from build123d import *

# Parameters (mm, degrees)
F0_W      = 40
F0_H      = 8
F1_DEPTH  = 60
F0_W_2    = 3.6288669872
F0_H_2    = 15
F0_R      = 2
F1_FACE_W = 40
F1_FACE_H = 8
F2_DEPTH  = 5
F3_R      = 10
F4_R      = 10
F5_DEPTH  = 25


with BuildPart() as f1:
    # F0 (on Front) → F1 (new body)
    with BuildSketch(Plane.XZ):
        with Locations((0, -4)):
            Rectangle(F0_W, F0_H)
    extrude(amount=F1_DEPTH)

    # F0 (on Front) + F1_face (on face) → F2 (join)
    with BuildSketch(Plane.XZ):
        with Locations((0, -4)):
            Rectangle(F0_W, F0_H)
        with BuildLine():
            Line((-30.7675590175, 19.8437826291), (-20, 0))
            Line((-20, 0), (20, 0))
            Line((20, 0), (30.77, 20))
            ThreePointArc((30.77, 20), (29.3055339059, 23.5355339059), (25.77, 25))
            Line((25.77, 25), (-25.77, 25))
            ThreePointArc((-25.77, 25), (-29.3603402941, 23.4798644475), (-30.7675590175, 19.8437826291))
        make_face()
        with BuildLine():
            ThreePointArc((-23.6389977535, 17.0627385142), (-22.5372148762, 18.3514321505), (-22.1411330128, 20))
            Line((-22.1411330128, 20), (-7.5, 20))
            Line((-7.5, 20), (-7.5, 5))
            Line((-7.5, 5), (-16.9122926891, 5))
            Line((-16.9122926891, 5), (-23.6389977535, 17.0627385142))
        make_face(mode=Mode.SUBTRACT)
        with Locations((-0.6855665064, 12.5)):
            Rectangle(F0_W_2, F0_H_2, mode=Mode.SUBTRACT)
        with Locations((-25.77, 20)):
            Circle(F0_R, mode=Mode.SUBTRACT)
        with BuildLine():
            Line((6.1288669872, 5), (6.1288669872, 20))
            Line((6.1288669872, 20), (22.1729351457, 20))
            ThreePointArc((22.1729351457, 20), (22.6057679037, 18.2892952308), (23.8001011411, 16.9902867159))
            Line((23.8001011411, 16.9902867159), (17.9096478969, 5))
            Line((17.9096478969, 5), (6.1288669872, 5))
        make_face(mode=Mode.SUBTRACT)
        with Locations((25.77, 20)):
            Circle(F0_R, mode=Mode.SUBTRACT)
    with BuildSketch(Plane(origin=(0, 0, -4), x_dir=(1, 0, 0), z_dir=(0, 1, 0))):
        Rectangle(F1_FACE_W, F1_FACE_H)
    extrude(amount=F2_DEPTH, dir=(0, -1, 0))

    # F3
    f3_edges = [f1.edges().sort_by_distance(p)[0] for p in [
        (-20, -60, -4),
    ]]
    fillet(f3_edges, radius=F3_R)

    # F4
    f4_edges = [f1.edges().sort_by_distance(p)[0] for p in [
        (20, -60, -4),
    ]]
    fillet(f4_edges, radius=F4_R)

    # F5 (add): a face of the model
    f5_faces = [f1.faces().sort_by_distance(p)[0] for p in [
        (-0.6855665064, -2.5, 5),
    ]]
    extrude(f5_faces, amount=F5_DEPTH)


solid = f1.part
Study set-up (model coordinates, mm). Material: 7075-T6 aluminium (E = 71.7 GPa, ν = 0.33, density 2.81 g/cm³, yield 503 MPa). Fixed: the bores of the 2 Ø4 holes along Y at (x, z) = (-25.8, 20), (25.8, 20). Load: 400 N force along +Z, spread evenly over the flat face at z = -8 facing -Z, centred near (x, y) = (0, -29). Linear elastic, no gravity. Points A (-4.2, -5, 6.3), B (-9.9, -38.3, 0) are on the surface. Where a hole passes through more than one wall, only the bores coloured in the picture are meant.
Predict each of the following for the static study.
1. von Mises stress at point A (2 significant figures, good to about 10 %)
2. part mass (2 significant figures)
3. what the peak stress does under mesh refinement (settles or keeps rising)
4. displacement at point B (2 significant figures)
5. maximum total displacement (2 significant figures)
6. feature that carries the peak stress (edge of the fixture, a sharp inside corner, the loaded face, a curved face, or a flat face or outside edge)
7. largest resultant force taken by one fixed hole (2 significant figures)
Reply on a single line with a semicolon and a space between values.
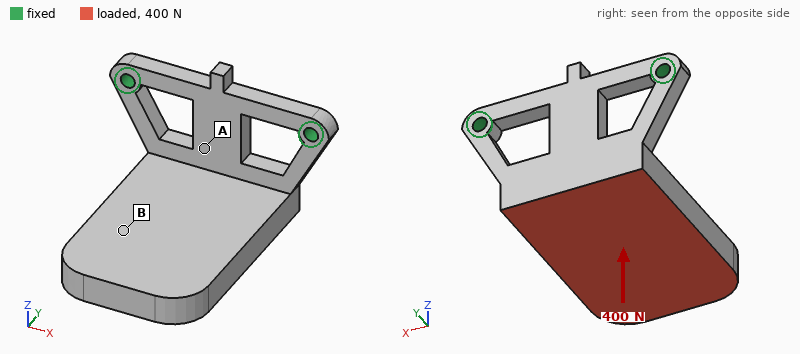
99 MPa; 65 g; keeps rising; 0.65 mm; 1.1 mm; edge of the fixture; 220 N
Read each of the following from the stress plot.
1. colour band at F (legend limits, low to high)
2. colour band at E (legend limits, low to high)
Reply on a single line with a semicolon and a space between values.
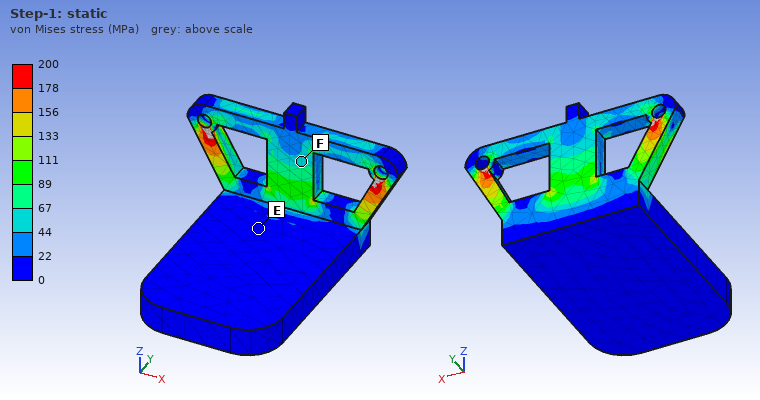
44 to 67 MPa; 0 to 22 MPa
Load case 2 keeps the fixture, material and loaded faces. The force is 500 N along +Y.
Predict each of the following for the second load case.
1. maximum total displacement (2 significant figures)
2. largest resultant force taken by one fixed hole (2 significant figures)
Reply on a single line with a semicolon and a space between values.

0.91 mm; 250 N
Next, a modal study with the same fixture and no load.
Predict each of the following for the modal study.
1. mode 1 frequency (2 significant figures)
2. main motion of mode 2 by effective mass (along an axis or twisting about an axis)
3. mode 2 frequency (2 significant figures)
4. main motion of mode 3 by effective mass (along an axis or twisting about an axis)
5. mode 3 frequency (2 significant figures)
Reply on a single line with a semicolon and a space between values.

490 Hz; along X; 1300 Hz; along Y; 2100 Hz
